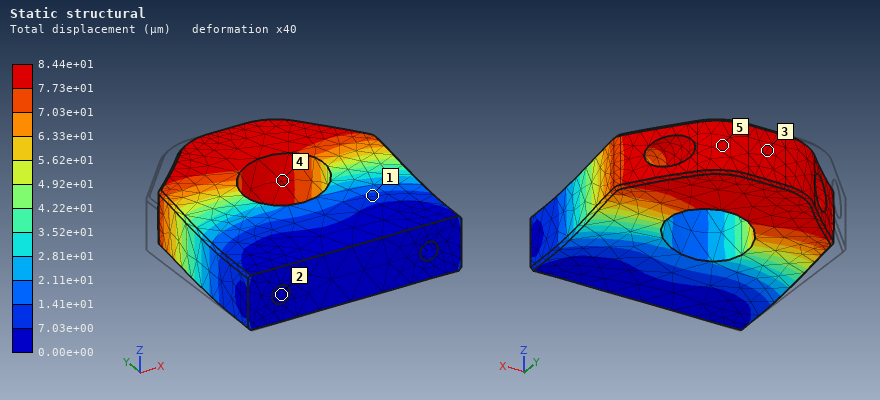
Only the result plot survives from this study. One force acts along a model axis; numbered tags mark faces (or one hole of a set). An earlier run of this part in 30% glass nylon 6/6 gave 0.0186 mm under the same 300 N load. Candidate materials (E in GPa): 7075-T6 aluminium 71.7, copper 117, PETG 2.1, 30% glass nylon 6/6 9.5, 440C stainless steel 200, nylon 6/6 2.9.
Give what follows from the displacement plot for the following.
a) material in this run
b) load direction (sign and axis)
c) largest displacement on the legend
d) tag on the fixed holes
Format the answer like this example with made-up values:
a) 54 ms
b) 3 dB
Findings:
a) PETG
b) +X
c) 8.44e+01 µm
d) 2
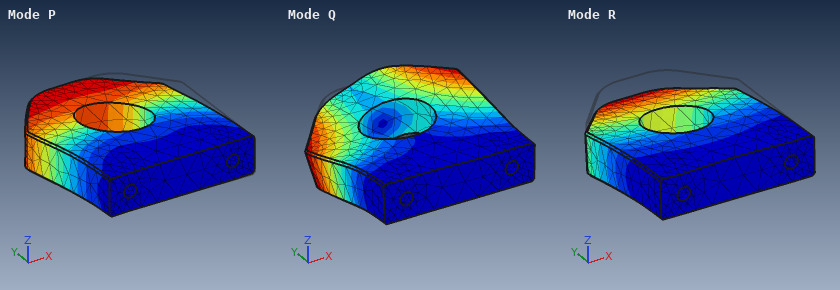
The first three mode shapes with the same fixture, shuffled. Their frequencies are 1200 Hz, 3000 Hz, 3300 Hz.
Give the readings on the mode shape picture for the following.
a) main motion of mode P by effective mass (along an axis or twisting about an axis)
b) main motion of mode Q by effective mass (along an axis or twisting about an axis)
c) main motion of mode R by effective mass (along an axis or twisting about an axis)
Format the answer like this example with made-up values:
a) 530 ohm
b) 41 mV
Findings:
a) along X
b) twisting about Y
c) along Z
